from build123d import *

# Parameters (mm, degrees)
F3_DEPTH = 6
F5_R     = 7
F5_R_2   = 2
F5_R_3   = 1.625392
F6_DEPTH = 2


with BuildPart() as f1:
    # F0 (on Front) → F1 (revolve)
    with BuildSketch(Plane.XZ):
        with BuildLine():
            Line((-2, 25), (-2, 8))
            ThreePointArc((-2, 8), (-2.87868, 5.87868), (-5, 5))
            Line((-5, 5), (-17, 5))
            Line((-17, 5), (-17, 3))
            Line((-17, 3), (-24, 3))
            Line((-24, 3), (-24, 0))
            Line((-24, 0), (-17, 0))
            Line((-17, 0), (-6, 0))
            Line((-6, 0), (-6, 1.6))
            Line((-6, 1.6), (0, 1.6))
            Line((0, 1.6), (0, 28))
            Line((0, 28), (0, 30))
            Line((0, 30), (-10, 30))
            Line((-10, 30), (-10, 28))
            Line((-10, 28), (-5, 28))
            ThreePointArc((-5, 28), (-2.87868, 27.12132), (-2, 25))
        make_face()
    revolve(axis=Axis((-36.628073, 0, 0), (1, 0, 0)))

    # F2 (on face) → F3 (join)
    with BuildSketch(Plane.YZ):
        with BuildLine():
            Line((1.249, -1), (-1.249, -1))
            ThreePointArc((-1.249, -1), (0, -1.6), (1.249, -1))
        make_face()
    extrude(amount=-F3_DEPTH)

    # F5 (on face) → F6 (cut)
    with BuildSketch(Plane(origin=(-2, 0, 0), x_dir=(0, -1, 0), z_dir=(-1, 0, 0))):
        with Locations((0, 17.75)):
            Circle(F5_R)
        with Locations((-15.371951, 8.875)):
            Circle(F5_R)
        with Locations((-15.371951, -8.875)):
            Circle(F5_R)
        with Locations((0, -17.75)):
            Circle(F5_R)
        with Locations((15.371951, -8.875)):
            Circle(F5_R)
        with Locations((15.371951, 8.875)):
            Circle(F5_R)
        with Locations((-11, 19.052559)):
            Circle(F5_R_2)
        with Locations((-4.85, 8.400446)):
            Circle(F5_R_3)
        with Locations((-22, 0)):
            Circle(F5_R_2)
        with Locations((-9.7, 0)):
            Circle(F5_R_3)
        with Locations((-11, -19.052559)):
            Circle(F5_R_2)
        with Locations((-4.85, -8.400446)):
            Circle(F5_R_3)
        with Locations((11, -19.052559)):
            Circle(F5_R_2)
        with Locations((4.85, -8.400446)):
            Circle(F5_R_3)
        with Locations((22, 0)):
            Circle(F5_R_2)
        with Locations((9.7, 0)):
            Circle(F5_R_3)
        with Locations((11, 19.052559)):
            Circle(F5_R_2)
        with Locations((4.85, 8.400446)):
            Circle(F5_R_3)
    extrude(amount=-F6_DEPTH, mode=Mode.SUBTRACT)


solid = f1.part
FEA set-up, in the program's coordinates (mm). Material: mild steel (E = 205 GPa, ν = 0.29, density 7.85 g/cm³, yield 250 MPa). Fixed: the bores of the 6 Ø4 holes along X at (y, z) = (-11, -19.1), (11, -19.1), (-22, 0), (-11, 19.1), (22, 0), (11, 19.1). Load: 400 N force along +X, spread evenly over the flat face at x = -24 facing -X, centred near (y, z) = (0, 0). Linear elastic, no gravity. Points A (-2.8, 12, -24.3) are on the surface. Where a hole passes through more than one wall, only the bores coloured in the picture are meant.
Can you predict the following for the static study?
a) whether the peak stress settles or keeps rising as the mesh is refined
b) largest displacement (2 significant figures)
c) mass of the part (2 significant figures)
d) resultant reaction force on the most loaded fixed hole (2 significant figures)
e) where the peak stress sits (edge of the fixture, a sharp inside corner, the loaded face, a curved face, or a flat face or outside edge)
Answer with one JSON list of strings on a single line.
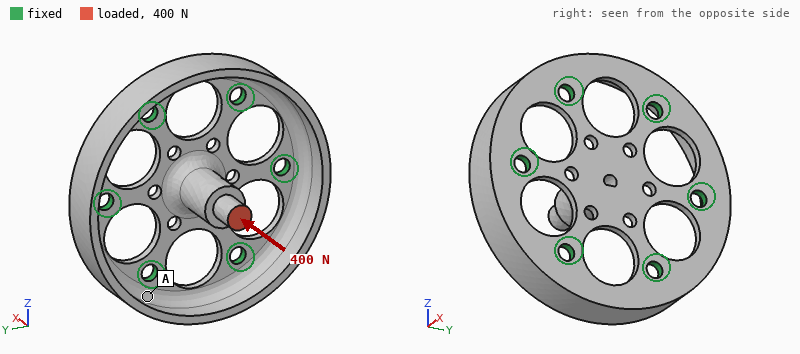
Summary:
["keeps rising", "24 µm", "64 g", "70 N", "edge of the fixture"]
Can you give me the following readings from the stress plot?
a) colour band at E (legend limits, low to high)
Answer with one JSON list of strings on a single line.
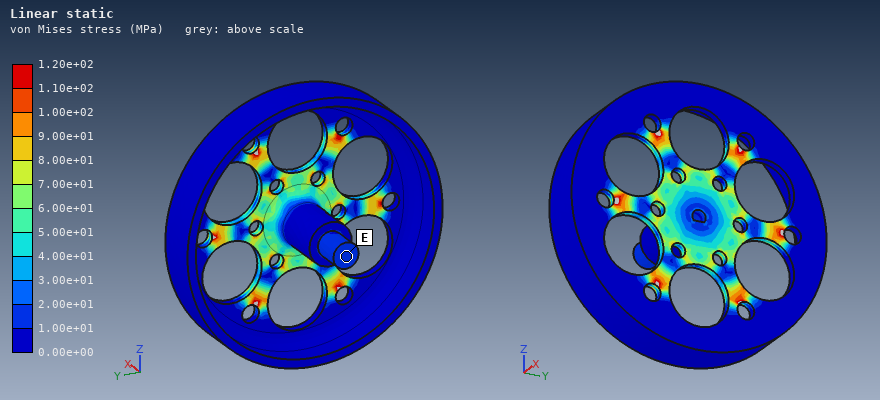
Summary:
["1.00e+01 to 2.00e+01 MPa"]
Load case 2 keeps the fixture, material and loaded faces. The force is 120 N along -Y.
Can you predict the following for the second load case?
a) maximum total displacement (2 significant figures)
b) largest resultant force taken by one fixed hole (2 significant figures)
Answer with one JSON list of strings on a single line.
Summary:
["41 µm", "70 N"]
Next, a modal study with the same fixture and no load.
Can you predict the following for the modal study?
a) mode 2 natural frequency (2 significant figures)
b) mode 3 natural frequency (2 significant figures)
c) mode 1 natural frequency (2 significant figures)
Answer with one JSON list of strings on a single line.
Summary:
["5200 Hz", "5200 Hz", "5200 Hz"]
